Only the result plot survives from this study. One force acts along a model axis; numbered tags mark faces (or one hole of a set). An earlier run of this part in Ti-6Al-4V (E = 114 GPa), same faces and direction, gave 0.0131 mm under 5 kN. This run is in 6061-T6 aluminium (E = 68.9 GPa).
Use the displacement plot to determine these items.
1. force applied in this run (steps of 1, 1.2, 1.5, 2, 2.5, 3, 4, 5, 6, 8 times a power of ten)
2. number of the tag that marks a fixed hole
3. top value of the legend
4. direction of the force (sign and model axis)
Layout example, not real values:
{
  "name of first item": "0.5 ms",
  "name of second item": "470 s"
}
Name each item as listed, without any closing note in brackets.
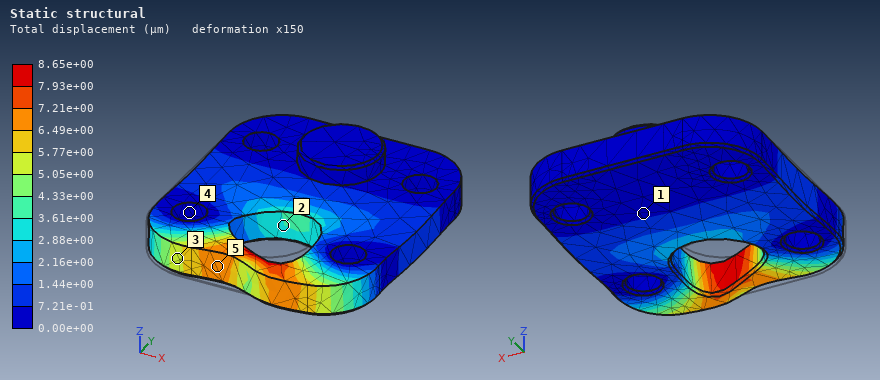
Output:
{
  "force applied in this run": "2 kN",
  "number of the tag that marks a fixed hole": "4",
  "top value of the legend": "8.65e+00 µm",
  "direction of the force": "+X"
}
